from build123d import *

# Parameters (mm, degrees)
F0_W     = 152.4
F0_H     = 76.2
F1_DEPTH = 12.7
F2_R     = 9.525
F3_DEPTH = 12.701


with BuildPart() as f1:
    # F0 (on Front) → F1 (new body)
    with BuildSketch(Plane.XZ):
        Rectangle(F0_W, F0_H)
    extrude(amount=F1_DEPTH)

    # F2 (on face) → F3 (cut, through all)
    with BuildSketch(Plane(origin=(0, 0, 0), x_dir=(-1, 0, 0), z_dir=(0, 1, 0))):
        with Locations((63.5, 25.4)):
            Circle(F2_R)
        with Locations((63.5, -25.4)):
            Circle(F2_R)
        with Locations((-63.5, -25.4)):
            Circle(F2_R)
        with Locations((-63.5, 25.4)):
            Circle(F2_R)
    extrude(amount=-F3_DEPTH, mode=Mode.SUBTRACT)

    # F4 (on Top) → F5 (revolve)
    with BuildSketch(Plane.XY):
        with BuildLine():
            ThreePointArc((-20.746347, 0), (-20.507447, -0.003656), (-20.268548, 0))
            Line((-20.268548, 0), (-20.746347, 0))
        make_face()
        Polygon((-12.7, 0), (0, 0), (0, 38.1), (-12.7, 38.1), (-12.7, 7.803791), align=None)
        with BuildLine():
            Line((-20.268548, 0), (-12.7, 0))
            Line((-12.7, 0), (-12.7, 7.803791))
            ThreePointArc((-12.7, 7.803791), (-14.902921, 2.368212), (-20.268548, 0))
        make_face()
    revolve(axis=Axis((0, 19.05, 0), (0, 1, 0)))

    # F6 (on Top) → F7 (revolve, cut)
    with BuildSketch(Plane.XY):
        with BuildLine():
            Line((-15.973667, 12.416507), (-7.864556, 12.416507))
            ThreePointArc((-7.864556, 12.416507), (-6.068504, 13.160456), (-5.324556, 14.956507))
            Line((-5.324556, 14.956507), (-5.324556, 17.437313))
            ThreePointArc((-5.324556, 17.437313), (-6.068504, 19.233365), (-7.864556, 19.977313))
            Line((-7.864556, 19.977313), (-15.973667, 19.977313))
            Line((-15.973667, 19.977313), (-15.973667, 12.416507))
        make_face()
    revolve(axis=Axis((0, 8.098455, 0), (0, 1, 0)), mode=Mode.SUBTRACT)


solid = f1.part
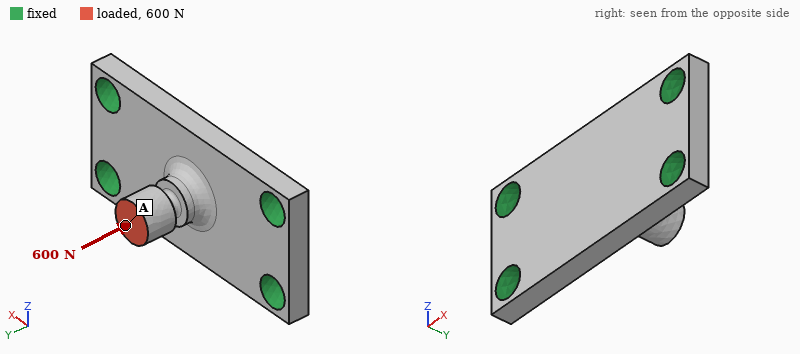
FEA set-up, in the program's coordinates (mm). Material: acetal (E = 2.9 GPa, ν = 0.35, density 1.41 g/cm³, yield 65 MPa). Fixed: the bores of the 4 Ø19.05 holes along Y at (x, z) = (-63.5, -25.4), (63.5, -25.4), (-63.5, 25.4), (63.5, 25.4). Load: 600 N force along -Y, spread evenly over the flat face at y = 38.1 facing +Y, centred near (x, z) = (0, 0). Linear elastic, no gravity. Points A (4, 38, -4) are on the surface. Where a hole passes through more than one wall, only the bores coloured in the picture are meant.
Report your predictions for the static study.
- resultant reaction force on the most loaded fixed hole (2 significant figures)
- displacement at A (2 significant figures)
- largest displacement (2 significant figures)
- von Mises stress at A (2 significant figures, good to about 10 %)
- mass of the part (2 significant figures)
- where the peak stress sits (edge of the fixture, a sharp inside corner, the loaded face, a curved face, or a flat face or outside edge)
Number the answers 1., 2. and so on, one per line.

1. 150 N
2. 0.14 mm
3. 0.14 mm
4. 1.4 MPa
5. 210 g
6. a curved face
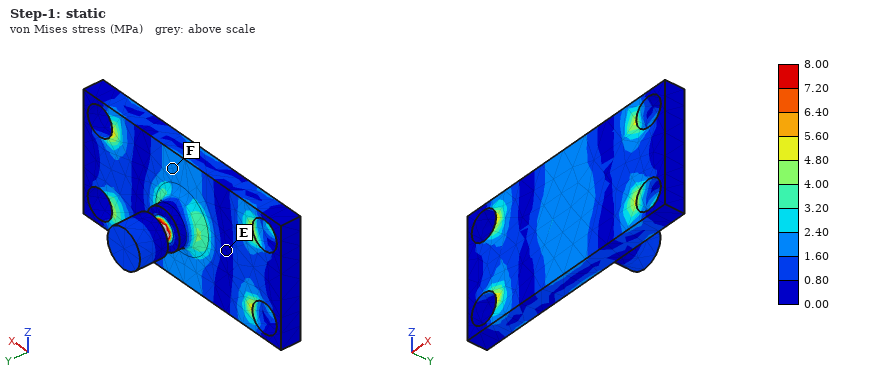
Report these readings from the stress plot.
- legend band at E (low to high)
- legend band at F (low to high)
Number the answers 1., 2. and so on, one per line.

1. 0.00 to 0.80 MPa
2. 1.60 to 2.40 MPa
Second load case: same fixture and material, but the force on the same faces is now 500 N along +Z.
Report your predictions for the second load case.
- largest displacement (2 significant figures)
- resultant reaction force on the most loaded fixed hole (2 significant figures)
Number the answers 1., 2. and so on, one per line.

1. 1.8 mm
2. 280 N
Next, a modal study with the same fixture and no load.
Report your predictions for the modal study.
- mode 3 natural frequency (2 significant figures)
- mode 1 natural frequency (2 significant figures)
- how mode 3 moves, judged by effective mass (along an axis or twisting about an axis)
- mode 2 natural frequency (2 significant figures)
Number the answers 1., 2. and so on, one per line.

1. 1200 Hz
2. 1000 Hz
3. along Y
4. 1100 Hz
